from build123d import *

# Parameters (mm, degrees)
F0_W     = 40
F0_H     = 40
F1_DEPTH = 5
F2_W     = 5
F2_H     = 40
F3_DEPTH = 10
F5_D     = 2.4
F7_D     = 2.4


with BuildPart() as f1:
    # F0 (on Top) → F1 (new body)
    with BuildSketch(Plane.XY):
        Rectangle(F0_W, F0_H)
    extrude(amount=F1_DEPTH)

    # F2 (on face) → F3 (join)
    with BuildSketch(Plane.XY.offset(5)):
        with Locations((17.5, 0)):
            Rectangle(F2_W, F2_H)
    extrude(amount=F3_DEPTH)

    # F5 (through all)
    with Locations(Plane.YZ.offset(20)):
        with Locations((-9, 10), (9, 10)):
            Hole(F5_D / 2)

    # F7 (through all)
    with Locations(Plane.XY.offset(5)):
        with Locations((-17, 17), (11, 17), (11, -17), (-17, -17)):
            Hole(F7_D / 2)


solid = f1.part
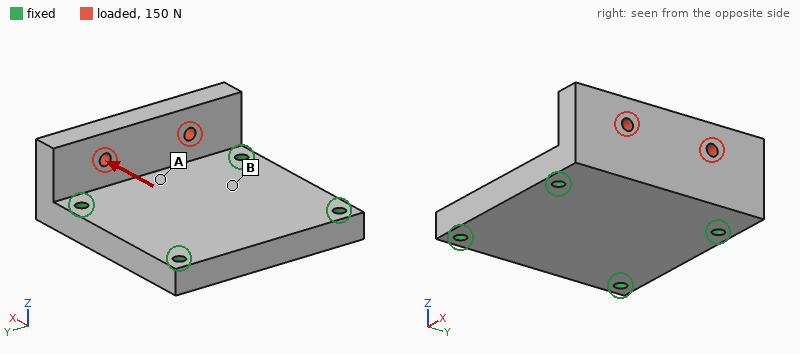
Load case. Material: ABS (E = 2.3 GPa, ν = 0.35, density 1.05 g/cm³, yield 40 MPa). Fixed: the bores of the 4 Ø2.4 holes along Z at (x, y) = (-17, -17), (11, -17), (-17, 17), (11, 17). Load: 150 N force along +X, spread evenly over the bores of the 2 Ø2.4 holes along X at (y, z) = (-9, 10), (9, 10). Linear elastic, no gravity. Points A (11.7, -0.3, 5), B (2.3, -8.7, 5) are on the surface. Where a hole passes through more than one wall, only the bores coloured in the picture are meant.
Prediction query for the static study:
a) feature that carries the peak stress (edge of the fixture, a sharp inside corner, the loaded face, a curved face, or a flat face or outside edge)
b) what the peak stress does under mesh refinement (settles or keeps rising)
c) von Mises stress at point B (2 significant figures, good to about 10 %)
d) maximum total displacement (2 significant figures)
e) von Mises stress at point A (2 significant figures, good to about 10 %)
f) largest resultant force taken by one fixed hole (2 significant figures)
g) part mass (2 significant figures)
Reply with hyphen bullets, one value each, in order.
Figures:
- edge of the fixture
- keeps rising
- 2.0 MPa
- 0.18 mm
- 4.9 MPa
- 52 N
- 10 g
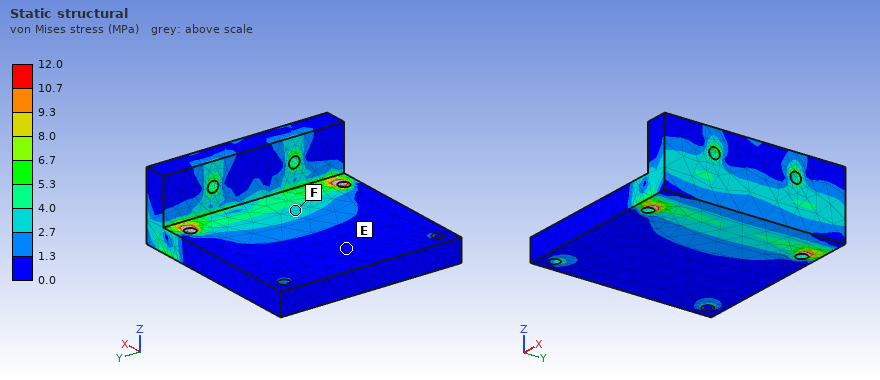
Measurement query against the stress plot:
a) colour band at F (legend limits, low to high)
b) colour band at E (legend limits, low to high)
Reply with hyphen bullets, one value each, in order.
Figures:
- 2.7 to 4.0 MPa
- 0.0 to 1.3 MPa
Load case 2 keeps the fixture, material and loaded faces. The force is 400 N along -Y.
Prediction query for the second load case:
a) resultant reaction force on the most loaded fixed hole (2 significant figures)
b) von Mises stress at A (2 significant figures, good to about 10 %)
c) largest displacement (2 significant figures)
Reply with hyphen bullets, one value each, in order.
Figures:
- 220 N
- 3.7 MPa
- 93 µm
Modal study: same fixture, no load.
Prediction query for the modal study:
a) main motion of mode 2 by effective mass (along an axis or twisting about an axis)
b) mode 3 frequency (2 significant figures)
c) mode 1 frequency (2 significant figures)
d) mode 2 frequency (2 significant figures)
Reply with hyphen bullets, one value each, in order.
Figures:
- along Z
- 5500 Hz
- 3400 Hz
- 4700 Hz
